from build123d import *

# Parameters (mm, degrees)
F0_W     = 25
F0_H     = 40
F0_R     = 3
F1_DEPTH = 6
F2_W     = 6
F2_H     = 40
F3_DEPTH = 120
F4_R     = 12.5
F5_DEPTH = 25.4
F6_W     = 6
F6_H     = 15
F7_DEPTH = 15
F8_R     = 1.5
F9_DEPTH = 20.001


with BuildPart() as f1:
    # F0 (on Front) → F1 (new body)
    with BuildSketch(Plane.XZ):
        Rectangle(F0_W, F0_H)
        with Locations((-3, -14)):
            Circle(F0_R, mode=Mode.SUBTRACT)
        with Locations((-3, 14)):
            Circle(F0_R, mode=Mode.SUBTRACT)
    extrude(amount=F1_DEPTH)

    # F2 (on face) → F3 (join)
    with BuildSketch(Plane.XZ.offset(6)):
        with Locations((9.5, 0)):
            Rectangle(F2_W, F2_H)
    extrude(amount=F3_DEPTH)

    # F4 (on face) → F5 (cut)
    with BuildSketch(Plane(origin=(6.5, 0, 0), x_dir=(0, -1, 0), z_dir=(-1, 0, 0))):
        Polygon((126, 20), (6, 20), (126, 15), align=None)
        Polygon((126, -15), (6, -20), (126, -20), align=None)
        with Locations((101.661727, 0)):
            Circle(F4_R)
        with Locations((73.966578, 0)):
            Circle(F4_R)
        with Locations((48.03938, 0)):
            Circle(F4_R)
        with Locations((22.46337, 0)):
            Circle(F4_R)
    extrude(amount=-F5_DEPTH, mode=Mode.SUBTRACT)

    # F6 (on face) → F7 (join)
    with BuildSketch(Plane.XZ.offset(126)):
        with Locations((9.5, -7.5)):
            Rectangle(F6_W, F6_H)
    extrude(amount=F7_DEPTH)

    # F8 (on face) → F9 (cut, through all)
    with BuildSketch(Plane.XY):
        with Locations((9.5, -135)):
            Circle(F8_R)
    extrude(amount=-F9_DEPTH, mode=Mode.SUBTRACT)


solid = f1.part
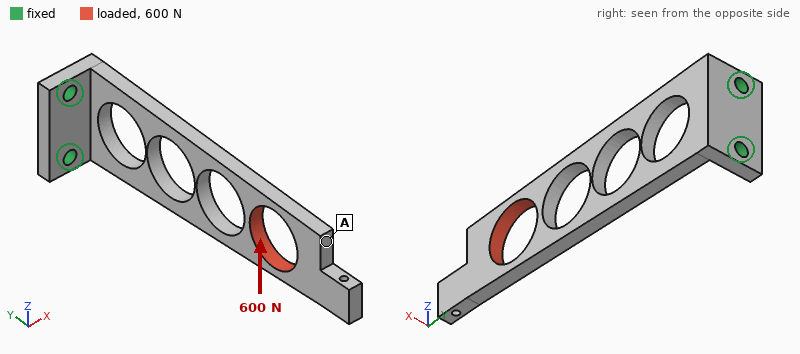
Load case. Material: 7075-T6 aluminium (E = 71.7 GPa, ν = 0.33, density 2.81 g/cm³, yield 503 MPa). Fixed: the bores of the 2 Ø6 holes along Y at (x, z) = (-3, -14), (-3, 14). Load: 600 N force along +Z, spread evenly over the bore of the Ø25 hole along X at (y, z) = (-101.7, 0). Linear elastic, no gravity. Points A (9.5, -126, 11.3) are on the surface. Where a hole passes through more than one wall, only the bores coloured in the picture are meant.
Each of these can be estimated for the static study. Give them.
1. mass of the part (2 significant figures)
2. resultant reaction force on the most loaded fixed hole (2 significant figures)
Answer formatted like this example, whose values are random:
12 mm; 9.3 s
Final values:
57 g; 2.0 kN
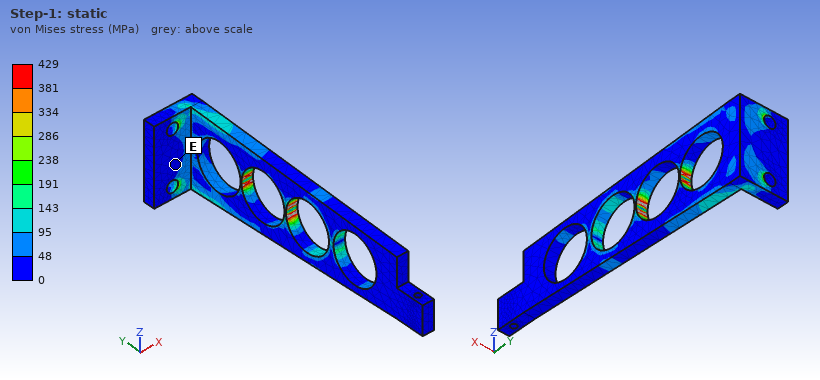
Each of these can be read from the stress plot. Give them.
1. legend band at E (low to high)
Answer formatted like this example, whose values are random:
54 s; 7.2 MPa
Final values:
0 to 48 MPa
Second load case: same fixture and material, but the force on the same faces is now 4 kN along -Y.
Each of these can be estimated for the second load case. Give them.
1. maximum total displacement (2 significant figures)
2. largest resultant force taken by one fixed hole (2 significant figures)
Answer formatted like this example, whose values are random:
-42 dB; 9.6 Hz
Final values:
0.77 mm; 2.0 kN
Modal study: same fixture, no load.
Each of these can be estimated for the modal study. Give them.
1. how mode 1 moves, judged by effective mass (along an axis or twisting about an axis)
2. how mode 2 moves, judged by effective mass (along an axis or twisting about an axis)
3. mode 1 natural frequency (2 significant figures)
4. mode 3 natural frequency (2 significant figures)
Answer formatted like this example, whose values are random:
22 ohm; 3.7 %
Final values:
along X; along Z; 240 Hz; 1300 Hz
